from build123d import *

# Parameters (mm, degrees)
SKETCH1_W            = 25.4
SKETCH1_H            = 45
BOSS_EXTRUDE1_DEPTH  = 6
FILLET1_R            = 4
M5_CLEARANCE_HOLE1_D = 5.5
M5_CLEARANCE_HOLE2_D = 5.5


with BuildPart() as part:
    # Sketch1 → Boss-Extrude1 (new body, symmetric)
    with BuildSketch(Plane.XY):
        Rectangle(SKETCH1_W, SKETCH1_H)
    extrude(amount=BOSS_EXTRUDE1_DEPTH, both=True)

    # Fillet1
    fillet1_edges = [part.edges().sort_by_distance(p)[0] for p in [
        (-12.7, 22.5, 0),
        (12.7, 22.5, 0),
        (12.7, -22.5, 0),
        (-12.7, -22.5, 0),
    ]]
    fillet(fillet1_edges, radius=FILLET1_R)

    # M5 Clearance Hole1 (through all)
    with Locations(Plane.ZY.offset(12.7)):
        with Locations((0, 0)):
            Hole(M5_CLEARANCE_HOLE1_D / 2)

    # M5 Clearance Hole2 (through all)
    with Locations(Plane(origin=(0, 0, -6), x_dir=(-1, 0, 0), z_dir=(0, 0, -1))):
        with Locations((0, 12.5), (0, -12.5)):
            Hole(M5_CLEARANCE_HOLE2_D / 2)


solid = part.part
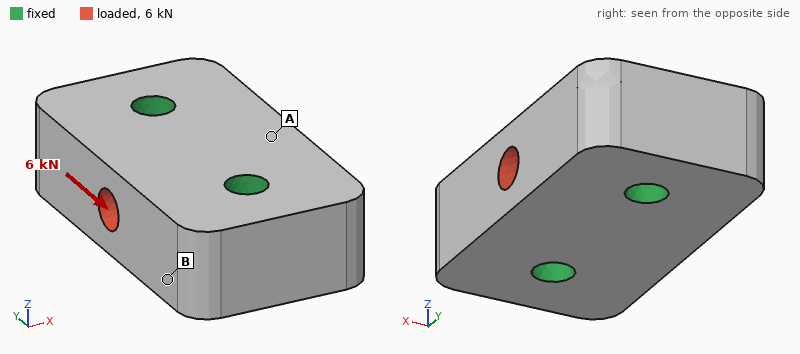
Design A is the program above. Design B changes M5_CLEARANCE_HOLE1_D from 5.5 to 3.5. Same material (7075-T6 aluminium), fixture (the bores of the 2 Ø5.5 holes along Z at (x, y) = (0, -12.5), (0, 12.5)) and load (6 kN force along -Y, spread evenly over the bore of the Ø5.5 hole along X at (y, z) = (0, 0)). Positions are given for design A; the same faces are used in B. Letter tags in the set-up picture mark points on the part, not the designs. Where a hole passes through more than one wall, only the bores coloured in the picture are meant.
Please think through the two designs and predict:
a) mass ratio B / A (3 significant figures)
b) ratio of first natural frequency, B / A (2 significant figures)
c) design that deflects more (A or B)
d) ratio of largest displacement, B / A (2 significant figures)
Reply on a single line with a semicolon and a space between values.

1.03; 0.98; B; 1.1
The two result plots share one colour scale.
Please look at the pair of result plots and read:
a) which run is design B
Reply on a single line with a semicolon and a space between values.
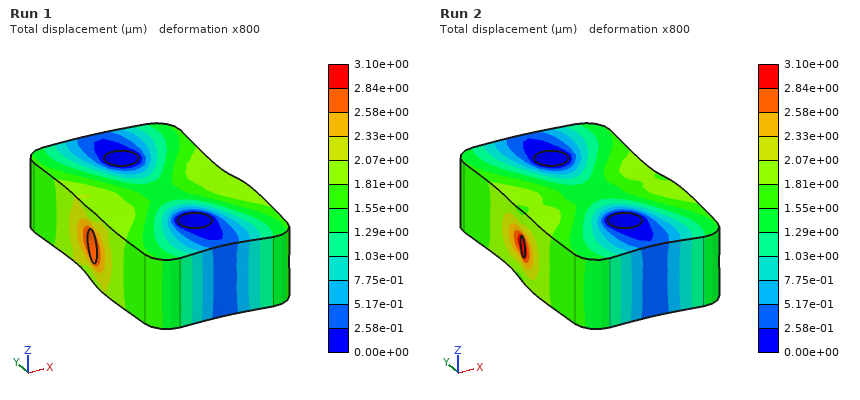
Run 2
